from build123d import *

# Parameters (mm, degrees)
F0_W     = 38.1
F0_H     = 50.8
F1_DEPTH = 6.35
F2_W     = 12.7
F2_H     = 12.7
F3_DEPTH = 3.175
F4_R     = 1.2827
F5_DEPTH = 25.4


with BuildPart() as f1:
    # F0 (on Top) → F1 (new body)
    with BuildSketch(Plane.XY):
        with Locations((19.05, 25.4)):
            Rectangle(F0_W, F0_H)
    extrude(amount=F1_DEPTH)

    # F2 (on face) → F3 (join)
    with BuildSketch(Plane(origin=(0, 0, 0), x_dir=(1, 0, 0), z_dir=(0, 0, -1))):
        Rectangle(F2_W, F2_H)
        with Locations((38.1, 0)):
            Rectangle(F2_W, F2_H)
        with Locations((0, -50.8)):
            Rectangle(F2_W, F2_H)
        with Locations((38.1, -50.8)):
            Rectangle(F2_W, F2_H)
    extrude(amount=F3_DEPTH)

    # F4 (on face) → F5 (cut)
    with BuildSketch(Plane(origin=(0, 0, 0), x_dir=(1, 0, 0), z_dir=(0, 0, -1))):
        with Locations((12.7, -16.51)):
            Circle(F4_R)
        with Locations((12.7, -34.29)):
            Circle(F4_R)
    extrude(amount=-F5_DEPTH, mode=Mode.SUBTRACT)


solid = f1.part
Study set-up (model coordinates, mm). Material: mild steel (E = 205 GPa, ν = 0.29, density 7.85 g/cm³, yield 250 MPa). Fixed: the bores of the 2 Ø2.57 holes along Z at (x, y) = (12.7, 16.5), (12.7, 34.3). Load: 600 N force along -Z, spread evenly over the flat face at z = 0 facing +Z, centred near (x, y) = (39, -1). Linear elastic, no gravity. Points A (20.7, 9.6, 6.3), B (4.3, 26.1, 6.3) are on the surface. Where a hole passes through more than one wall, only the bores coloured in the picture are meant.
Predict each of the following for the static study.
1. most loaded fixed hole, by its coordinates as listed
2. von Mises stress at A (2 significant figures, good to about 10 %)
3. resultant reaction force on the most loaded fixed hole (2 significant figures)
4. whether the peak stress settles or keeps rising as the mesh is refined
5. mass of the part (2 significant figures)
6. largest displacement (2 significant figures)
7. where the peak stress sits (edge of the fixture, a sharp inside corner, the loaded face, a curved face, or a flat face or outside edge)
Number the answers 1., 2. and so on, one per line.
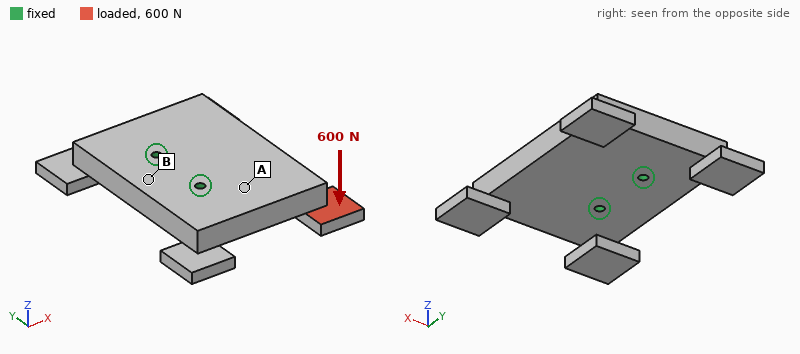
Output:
1. (12.7, 16.5)
2. 59 MPa
3. 910 N
4. keeps rising
5. 110 g
6. 0.11 mm
7. edge of the fixture
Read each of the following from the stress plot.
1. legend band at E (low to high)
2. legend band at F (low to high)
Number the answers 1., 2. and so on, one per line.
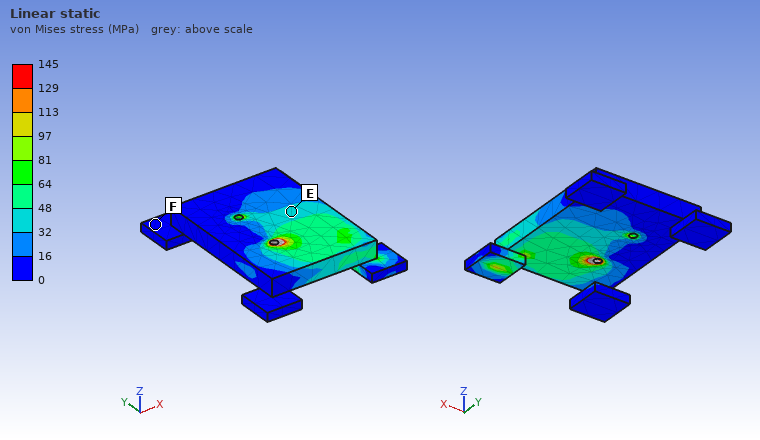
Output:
1. 32 to 48 MPa
2. 0 to 16 MPa
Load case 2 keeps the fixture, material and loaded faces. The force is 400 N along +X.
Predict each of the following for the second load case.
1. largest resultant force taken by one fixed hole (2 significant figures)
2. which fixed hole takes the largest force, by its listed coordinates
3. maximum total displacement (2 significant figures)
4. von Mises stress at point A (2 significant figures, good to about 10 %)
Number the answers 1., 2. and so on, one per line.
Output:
1. 760 N
2. (12.7, 16.5)
3. 10 µm
4. 4.1 MPa
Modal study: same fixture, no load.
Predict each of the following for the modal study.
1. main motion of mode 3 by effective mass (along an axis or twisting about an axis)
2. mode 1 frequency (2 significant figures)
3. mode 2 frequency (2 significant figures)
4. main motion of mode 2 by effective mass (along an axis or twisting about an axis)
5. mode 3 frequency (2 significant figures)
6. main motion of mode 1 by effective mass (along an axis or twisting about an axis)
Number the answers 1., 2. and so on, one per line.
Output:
1. along Z
2. 4800 Hz
3. 5800 Hz
4. twisting about X
5. 8800 Hz
6. along Z
